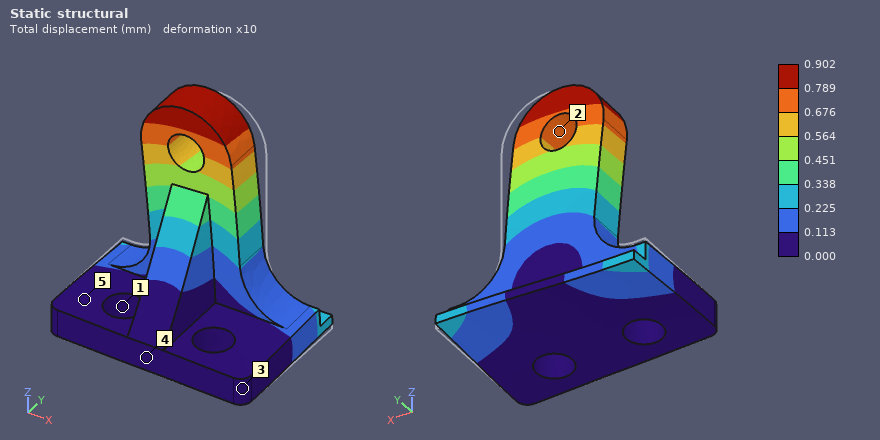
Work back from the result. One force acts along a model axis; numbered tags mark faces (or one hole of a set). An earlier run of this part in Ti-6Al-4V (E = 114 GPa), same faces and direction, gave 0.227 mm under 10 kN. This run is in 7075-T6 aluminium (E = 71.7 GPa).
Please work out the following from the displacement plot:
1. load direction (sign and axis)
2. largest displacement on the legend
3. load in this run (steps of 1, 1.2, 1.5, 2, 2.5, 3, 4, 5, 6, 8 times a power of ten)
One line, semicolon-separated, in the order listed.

-X; 0.902 mm; 25 kN
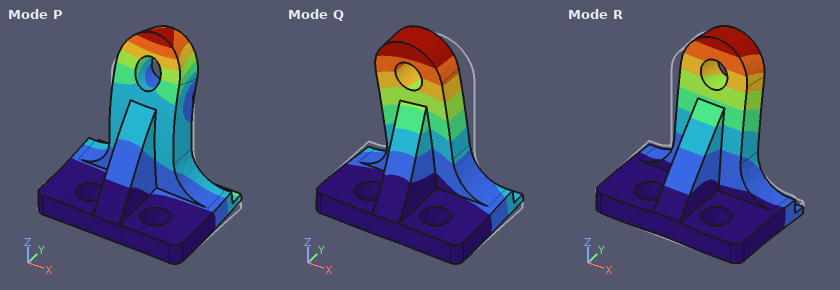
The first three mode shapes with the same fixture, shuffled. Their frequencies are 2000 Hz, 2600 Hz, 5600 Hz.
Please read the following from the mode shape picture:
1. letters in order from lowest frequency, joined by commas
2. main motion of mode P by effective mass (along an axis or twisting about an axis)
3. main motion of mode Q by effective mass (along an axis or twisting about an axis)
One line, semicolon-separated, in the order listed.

R, Q, P; along Z; along X
